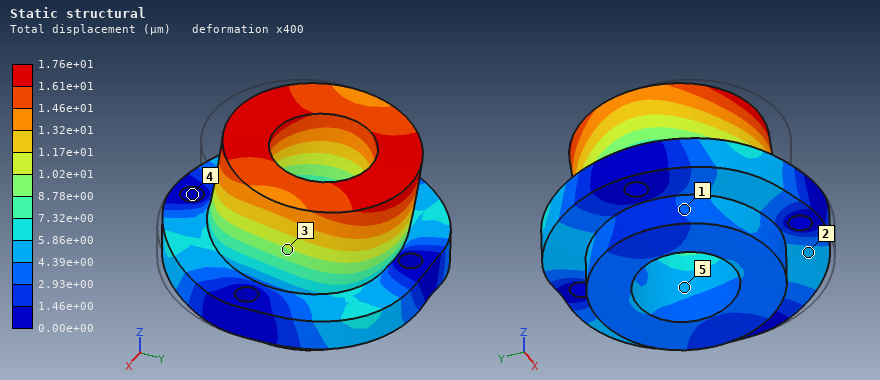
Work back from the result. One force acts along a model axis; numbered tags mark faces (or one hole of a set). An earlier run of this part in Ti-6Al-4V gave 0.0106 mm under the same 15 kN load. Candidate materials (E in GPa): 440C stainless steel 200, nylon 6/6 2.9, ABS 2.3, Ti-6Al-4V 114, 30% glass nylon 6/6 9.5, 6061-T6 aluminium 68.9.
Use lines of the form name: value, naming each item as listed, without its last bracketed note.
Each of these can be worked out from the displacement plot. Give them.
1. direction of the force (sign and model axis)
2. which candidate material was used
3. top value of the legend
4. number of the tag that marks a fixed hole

direction of the force: +Y
which candidate material was used: 6061-T6 aluminium
top value of the legend: 1.76e+01 µm
number of the tag that marks a fixed hole: 4
